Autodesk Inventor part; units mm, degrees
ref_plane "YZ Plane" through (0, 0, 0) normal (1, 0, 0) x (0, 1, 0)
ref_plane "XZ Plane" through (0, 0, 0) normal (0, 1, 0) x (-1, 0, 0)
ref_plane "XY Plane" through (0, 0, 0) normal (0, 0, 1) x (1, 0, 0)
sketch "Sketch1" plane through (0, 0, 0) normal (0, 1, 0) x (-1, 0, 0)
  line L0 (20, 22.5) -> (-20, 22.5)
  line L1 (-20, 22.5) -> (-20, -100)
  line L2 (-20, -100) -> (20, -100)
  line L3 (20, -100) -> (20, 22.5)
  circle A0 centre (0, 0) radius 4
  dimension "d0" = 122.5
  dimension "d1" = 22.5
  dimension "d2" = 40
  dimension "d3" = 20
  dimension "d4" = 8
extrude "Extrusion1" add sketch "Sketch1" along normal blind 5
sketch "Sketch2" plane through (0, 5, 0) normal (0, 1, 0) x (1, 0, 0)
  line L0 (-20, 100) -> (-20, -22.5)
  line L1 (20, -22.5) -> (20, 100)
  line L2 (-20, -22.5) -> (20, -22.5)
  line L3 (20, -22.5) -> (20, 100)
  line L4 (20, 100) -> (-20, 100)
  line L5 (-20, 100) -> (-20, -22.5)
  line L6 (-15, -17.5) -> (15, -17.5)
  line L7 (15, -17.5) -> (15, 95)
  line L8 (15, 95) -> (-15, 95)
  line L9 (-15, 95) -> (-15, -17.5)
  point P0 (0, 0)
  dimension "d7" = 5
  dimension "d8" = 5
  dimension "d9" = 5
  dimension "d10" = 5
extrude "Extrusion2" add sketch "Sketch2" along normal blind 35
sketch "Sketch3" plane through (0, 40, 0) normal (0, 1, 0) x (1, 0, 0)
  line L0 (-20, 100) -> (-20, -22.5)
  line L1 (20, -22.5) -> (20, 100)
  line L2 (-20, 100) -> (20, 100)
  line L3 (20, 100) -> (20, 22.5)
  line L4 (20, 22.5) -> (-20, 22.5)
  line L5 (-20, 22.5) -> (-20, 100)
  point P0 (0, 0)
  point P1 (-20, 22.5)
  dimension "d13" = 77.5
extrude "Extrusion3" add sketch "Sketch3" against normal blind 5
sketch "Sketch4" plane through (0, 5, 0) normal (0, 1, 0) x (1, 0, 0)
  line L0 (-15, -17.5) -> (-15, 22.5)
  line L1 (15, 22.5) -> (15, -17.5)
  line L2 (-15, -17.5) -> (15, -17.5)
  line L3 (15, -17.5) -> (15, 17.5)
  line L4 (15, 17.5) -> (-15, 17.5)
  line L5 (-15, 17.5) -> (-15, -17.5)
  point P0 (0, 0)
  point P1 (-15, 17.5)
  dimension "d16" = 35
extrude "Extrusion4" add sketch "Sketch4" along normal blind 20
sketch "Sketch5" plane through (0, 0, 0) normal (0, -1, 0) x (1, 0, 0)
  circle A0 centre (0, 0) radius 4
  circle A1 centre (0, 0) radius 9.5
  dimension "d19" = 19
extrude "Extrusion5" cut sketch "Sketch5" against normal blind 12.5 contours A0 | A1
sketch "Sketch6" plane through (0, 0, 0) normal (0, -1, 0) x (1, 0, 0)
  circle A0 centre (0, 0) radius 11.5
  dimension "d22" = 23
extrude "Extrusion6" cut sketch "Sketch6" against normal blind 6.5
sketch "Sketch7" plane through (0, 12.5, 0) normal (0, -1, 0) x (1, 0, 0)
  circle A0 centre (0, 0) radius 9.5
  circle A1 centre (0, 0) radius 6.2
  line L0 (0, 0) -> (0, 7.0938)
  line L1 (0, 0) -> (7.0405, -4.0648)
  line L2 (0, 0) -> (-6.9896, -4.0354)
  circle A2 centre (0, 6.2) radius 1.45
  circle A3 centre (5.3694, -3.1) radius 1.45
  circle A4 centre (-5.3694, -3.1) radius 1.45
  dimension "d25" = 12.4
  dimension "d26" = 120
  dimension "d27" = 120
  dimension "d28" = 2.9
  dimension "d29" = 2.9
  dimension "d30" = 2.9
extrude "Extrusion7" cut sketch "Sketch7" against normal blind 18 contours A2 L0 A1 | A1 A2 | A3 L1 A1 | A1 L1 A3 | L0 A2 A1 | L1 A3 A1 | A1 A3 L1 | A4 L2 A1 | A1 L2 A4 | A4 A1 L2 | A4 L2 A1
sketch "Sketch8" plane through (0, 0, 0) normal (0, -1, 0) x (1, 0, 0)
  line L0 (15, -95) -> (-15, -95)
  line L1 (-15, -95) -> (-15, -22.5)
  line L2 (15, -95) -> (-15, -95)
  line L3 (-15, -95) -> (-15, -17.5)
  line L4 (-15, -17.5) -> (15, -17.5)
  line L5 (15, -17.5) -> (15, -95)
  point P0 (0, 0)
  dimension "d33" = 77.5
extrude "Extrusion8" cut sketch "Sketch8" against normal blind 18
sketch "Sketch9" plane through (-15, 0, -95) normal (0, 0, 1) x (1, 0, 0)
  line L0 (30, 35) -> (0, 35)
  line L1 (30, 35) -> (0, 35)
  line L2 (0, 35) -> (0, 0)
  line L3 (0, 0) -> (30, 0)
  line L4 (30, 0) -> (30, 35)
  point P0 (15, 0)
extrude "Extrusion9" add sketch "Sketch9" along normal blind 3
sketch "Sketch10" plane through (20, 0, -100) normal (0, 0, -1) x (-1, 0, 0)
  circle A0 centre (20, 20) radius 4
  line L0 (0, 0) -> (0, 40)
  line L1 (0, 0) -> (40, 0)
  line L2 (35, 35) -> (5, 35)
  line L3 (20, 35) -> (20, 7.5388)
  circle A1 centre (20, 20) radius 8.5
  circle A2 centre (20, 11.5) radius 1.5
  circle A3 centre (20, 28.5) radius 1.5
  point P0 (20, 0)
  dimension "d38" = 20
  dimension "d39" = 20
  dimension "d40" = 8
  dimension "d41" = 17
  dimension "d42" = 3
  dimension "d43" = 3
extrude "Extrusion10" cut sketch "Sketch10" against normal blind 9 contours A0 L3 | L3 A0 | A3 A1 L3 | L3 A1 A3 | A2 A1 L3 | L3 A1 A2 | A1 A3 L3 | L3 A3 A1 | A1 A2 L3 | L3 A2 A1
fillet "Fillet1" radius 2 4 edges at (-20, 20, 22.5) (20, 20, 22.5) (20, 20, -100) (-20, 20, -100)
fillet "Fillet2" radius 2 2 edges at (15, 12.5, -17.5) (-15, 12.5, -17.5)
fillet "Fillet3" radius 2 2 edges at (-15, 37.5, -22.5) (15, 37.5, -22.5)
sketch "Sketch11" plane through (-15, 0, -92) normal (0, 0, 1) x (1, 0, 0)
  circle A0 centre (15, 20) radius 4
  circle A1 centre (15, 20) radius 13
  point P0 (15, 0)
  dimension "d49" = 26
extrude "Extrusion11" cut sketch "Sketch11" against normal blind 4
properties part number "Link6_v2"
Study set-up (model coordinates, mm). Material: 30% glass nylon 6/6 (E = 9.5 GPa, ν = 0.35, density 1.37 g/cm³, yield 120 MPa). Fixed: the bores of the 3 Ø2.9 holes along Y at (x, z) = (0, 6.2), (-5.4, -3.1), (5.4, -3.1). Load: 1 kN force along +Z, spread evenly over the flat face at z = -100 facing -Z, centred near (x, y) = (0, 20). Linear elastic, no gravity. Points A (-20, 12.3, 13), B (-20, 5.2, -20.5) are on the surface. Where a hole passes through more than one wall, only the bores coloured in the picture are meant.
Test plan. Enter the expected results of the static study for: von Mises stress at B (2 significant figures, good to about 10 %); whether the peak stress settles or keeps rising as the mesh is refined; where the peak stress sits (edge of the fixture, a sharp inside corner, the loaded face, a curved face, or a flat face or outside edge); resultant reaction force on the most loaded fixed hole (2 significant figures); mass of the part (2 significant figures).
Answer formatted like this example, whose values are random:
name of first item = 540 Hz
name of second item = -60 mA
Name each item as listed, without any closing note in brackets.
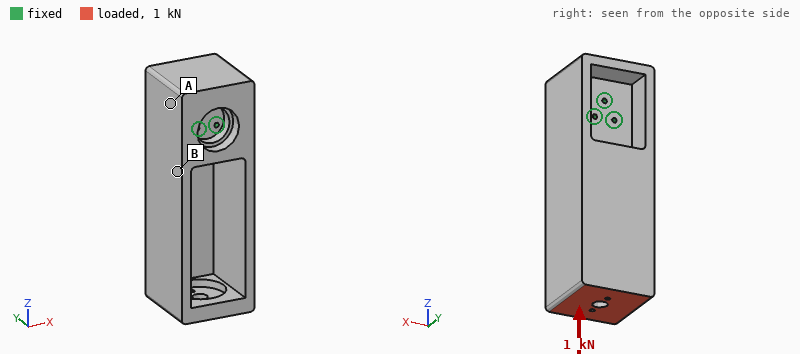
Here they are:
von Mises stress at B = 2.8 MPa
whether the peak stress settles or keeps rising as the mesh is refined = keeps rising
where the peak stress sits = a sharp inside corner
resultant reaction force on the most loaded fixed hole = 360 N
mass of the part = 130 g
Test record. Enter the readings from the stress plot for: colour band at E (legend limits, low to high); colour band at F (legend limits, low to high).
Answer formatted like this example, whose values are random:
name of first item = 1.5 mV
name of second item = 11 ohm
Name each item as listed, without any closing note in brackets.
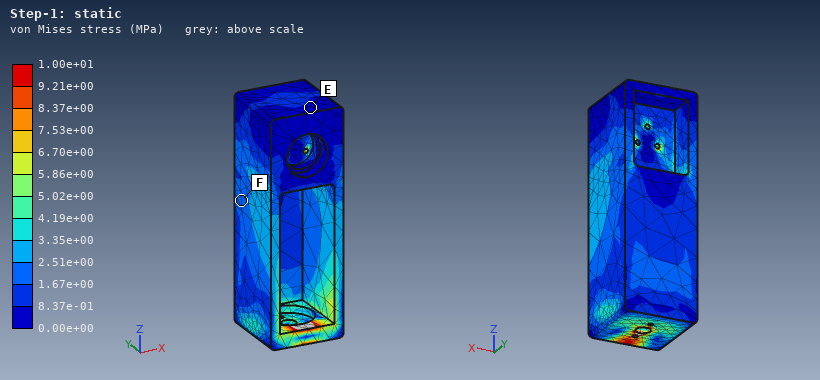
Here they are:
colour band at E = 0.00e+00 to 8.37e-01 MPa
colour band at F = 1.67e+00 to 2.51e+00 MPa
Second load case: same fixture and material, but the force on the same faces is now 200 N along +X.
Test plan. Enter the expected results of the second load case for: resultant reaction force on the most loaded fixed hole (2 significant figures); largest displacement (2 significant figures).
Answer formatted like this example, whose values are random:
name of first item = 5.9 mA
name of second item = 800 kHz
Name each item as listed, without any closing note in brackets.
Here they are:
resultant reaction force on the most loaded fixed hole = 1.0 kN
largest displacement = 0.53 mm
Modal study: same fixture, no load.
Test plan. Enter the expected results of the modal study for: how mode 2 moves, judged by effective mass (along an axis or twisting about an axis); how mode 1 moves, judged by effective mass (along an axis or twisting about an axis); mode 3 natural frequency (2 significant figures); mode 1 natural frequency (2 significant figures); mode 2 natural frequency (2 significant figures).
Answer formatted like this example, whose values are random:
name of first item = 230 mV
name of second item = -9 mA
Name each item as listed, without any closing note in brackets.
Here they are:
how mode 2 moves, judged by effective mass = along Y
how mode 1 moves, judged by effective mass = along X
mode 3 natural frequency = 1500 Hz
mode 1 natural frequency = 620 Hz
mode 2 natural frequency = 790 Hz
